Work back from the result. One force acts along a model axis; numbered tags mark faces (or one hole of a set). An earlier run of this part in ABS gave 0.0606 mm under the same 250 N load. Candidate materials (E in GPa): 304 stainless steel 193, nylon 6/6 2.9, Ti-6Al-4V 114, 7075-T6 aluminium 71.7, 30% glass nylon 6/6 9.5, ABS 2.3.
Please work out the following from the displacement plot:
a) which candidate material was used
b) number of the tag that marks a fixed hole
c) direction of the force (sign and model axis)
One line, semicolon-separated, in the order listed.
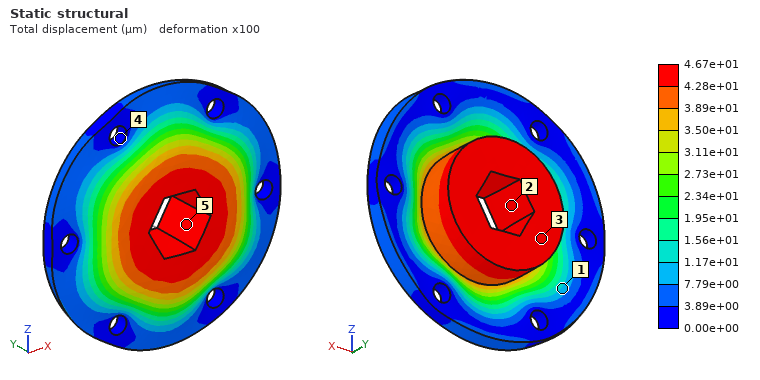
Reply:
nylon 6/6; 4; -Y
